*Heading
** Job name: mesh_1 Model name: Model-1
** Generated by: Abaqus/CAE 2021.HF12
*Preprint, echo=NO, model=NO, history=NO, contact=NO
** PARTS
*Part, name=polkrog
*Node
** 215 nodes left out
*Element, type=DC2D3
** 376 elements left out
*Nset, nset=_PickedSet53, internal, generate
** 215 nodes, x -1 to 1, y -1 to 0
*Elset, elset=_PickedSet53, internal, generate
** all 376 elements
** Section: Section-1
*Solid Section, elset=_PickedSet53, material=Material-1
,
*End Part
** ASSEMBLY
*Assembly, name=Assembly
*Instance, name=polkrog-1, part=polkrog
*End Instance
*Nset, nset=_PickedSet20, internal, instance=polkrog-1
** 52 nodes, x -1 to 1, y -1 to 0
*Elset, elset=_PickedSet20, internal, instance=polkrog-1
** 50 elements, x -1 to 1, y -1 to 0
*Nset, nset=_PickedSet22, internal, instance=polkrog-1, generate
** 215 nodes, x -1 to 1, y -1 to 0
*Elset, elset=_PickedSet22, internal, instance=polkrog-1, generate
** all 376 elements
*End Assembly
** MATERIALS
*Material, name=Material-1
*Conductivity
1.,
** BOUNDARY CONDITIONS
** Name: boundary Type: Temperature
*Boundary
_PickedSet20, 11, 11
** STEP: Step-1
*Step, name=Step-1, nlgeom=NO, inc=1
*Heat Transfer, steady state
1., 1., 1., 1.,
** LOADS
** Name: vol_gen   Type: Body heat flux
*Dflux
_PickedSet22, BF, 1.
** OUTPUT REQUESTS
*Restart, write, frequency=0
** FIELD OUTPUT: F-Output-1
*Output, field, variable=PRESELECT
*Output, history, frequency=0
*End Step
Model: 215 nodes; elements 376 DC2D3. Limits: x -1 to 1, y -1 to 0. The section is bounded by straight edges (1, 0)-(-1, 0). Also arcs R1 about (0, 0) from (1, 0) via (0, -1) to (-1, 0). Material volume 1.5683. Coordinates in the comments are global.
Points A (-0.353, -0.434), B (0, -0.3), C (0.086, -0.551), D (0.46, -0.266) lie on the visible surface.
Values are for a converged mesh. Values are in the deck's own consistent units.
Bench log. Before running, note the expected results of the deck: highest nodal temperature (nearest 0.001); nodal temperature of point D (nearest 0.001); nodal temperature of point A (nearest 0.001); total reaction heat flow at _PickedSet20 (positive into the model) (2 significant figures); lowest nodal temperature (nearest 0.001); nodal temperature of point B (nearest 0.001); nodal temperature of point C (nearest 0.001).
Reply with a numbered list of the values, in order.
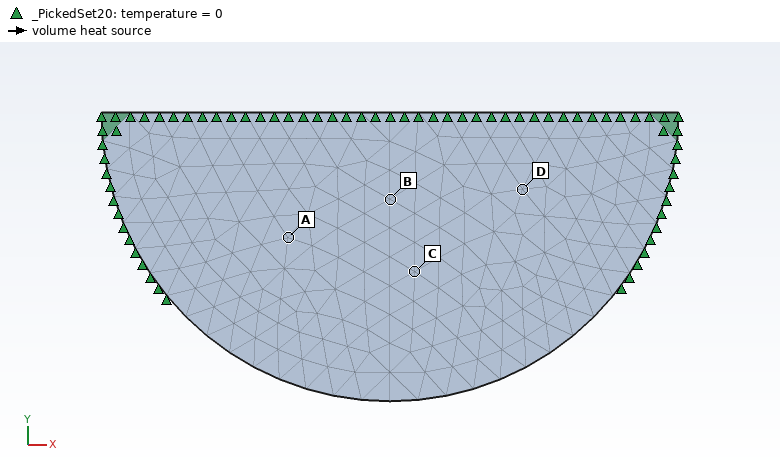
1. 0.097
2. 0.064
3. 0.084
4. -1.5
5. 0.000
6. 0.084
7. 0.095
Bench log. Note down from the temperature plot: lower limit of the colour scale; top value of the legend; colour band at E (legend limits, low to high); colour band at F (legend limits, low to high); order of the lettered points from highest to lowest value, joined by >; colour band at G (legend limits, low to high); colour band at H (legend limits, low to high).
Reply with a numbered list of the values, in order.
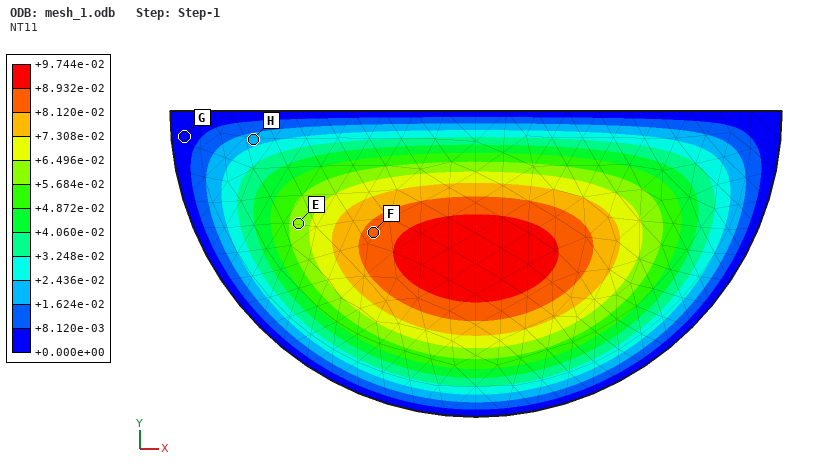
1. +0.000e+00
2. +9.744e-02
3. +5.684e-02 to +6.496e-02
4. +8.120e-02 to +8.932e-02
5. F > E > H > G
6. +0.000e+00 to +8.120e-03
7. +1.624e-02 to +2.436e-02
